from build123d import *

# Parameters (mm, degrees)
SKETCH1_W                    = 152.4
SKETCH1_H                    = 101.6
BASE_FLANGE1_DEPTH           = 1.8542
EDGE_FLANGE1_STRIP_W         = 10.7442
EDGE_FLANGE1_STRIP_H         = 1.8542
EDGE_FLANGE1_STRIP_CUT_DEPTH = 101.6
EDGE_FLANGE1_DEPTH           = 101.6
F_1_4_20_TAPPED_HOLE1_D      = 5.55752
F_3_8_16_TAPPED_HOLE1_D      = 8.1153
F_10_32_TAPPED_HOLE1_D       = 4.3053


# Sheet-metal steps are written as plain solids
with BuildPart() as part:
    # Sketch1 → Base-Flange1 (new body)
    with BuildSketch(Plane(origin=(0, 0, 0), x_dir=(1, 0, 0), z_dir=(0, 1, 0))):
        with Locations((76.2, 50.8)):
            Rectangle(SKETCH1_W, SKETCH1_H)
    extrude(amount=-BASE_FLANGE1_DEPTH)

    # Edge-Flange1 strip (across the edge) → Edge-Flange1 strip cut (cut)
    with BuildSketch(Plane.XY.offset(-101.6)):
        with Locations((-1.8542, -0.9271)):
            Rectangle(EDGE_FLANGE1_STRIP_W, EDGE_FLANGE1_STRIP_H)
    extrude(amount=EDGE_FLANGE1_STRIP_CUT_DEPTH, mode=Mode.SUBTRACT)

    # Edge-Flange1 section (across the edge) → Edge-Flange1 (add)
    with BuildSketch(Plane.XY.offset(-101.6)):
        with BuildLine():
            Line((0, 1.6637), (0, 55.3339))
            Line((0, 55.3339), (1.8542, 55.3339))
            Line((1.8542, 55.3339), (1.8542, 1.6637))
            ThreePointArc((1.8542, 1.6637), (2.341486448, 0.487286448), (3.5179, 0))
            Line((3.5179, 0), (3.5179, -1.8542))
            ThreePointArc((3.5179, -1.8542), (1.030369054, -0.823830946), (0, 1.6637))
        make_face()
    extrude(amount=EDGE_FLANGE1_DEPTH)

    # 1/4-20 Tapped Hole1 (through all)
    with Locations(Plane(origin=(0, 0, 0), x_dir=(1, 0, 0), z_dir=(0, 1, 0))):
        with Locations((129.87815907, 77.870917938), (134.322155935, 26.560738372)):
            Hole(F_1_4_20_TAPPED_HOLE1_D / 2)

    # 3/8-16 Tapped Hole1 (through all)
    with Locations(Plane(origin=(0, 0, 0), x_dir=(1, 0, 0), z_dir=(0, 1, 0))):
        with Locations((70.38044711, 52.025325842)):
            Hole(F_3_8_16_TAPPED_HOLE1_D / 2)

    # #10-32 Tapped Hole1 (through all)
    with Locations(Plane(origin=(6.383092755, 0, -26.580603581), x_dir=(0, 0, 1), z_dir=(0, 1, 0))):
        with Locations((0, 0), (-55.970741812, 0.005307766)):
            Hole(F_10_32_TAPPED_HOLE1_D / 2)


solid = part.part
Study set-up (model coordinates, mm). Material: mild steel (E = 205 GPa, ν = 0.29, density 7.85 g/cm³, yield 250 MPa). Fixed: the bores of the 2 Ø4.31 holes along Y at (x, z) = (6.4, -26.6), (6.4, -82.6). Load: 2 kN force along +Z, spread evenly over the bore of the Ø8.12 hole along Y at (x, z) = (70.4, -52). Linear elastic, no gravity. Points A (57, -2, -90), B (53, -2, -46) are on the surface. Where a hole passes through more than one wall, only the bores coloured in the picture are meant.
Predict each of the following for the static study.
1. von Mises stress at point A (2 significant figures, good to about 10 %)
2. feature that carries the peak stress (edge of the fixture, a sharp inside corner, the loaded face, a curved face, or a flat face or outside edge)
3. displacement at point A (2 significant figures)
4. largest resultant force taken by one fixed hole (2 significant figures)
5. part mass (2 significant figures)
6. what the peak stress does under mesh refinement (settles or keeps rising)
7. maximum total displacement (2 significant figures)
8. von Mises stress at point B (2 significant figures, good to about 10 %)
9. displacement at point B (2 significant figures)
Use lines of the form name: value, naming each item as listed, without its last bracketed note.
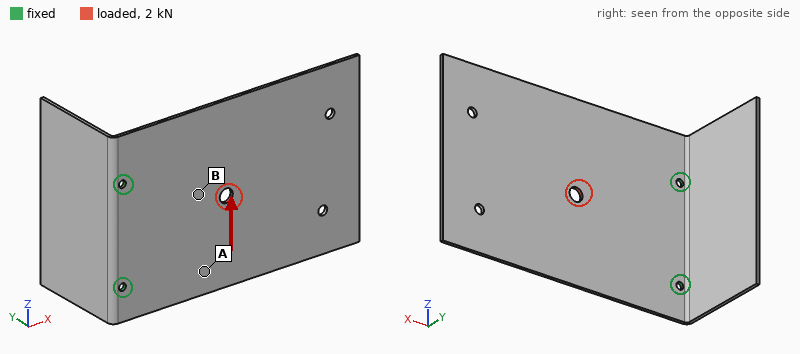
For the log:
von Mises stress at point A: 13 MPa
feature that carries the peak stress: edge of the fixture
displacement at point A: 24 µm
largest resultant force taken by one fixed hole: 2.4 kN
part mass: 300 g
what the peak stress does under mesh refinement: keeps rising
maximum total displacement: 54 µm
von Mises stress at point B: 30 MPa
displacement at point B: 20 µm
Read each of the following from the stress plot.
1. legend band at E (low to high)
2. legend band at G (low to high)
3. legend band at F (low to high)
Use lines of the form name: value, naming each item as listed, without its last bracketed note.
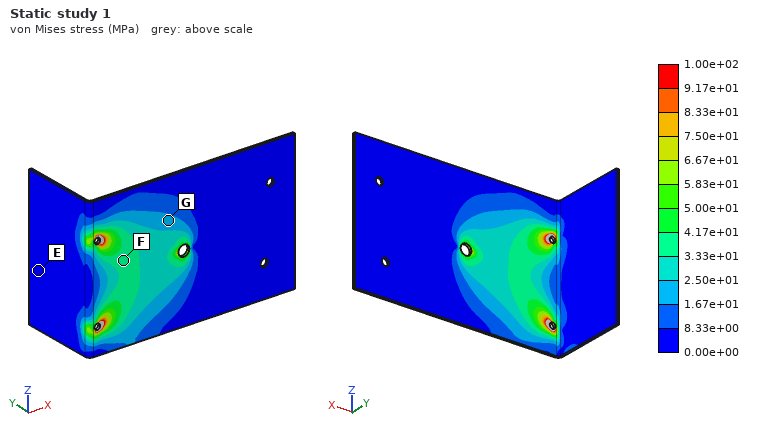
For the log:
legend band at E: 0.00e+00 to 8.33e+00 MPa
legend band at G: 1.67e+01 to 2.50e+01 MPa
legend band at F: 3.33e+01 to 4.17e+01 MPa
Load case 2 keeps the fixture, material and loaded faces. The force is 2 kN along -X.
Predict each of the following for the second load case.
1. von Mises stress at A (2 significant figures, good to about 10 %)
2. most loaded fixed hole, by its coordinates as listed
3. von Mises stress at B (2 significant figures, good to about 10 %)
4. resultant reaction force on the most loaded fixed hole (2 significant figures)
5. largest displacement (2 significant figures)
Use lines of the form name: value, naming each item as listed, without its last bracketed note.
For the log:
von Mises stress at A: 6.6 MPa
most loaded fixed hole, by its coordinates as listed: (6.4, -26.6)
von Mises stress at B: 21 MPa
resultant reaction force on the most loaded fixed hole: 1.1 kN
largest displacement: 8.0 µm
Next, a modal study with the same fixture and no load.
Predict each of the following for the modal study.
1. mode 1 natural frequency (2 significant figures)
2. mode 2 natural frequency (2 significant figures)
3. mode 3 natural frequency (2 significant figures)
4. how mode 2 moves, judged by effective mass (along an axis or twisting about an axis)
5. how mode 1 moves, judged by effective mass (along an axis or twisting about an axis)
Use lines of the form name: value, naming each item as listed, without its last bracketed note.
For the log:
mode 1 natural frequency: 71 Hz
mode 2 natural frequency: 230 Hz
mode 3 natural frequency: 390 Hz
how mode 2 moves, judged by effective mass: twisting about X
how mode 1 moves, judged by effective mass: along Y
